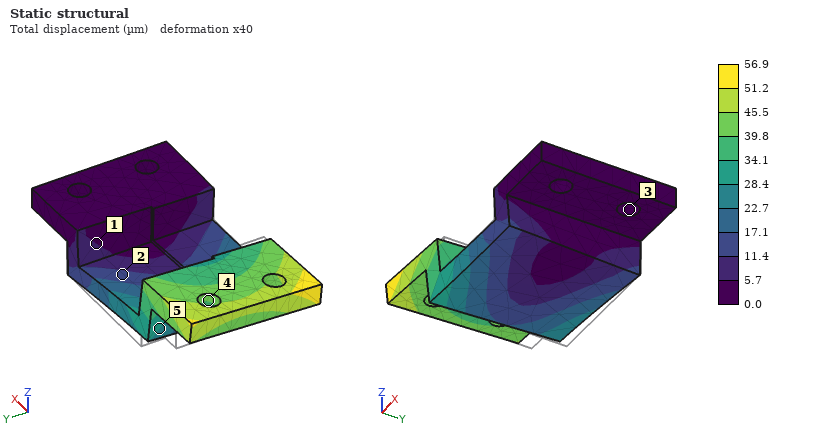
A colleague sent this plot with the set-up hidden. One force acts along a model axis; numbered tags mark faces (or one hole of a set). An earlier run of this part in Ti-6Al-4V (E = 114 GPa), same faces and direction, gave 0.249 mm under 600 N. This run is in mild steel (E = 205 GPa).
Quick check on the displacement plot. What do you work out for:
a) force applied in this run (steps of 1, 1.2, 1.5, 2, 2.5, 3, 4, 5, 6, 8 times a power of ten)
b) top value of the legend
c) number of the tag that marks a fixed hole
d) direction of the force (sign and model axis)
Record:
250 N
56.9 µm
3
-Y
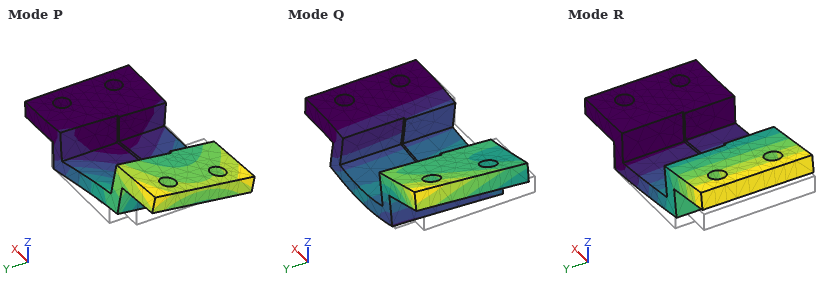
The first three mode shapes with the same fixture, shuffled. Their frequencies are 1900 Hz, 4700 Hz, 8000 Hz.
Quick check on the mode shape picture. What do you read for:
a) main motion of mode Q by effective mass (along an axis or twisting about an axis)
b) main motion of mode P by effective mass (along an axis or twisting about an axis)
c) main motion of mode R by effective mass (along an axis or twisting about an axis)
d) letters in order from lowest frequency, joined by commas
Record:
along X
along Y
along Z
R, P, Q
